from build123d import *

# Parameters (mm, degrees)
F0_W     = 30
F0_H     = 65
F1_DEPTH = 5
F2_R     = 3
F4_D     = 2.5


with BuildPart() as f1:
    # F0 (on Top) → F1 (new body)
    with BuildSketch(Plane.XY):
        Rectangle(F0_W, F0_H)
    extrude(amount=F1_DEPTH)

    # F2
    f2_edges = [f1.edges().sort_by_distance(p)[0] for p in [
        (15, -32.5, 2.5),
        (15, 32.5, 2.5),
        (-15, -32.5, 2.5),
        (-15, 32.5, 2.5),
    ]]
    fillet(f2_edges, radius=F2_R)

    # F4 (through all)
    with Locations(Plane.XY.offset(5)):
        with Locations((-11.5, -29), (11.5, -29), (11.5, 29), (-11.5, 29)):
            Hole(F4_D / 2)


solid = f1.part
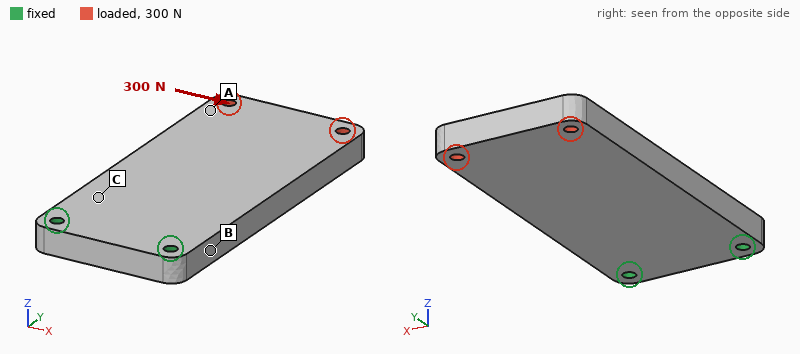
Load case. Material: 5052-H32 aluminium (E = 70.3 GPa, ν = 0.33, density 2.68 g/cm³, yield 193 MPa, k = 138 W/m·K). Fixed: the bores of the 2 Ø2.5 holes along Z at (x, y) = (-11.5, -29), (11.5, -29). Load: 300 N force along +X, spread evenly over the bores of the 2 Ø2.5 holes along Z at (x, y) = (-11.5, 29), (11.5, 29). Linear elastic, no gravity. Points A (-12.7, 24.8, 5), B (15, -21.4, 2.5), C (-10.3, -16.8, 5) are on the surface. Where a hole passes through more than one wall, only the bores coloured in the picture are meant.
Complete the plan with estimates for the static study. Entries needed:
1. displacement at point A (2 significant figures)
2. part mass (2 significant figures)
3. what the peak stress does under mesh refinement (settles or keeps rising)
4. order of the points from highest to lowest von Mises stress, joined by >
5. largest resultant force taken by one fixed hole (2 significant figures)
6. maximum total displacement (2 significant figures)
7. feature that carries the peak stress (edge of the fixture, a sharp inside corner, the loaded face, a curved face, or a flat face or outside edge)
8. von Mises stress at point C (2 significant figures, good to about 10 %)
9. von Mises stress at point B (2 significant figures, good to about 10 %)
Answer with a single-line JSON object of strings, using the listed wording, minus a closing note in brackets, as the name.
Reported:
{"displacement at point A": "29 µm", "part mass": "26 g", "what the peak stress does under mesh refinement": "keeps rising", "order of the points from highest to lowest von Mises stress, joined by >": "B > C > A", "largest resultant force taken by one fixed hole": "750 N", "maximum total displacement": "34 µm", "feature that carries the peak stress": "edge of the fixture", "von Mises stress at point C": "13 MPa", "von Mises stress at point B": "20 MPa"}
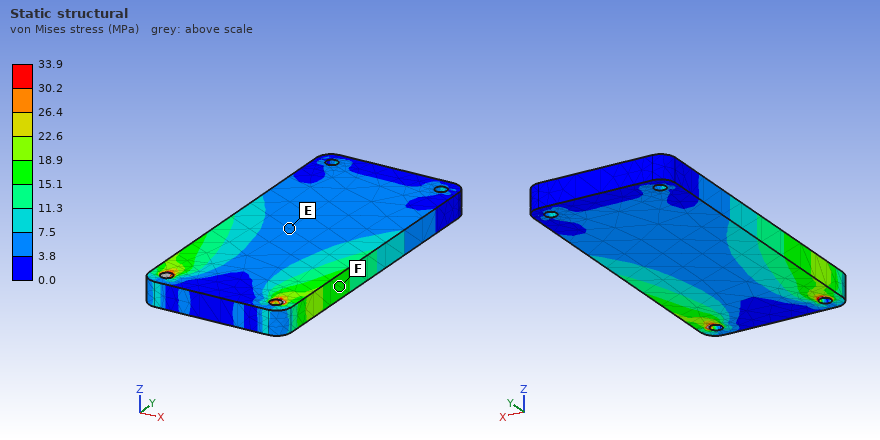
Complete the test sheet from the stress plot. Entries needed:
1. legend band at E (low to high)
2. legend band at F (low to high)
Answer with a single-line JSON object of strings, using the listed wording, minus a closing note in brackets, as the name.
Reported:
{"legend band at E": "3.8 to 7.5 MPa", "legend band at F": "15.1 to 18.9 MPa"}
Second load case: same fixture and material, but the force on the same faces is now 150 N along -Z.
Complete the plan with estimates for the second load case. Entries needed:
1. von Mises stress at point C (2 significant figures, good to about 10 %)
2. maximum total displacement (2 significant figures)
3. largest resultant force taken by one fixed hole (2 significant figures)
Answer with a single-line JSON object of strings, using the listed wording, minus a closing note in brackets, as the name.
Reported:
{"von Mises stress at point C": "56 MPa", "maximum total displacement": "0.55 mm", "largest resultant force taken by one fixed hole": "75 N"}
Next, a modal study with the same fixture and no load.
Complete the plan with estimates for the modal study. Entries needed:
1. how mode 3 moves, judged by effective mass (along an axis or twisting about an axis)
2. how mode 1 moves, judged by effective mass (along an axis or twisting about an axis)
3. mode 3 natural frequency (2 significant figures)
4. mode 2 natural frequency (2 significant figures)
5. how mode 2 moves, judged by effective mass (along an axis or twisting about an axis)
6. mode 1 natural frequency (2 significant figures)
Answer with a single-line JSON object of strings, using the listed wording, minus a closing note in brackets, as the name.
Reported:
{"how mode 3 moves, judged by effective mass": "along X", "how mode 1 moves, judged by effective mass": "along Z", "mode 3 natural frequency": "5600 Hz", "mode 2 natural frequency": "4600 Hz", "how mode 2 moves, judged by effective mass": "twisting about Y", "mode 1 natural frequency": "1000 Hz"}
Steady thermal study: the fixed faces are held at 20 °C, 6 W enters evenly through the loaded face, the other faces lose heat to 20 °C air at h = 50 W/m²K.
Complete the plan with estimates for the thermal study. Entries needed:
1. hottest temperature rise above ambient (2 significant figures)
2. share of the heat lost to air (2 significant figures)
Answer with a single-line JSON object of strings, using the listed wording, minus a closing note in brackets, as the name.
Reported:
{"hottest temperature rise above ambient": "16 K", "share of the heat lost to air": "28 %"}
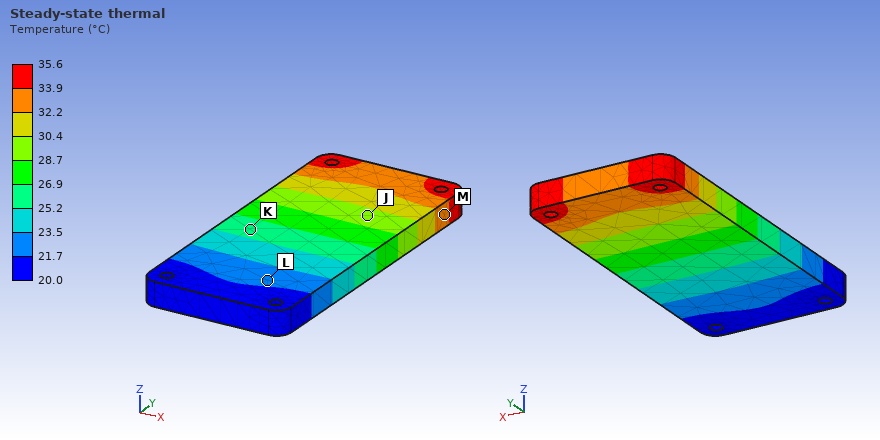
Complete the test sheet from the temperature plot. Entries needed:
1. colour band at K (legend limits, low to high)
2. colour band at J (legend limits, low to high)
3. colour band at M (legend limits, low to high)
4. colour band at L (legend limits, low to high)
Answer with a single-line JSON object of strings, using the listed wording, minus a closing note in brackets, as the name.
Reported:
{"colour band at K": "25.2 to 26.9 °C", "colour band at J": "28.7 to 30.4 °C", "colour band at M": "32.2 to 33.9 °C", "colour band at L": "21.7 to 23.5 °C"}
